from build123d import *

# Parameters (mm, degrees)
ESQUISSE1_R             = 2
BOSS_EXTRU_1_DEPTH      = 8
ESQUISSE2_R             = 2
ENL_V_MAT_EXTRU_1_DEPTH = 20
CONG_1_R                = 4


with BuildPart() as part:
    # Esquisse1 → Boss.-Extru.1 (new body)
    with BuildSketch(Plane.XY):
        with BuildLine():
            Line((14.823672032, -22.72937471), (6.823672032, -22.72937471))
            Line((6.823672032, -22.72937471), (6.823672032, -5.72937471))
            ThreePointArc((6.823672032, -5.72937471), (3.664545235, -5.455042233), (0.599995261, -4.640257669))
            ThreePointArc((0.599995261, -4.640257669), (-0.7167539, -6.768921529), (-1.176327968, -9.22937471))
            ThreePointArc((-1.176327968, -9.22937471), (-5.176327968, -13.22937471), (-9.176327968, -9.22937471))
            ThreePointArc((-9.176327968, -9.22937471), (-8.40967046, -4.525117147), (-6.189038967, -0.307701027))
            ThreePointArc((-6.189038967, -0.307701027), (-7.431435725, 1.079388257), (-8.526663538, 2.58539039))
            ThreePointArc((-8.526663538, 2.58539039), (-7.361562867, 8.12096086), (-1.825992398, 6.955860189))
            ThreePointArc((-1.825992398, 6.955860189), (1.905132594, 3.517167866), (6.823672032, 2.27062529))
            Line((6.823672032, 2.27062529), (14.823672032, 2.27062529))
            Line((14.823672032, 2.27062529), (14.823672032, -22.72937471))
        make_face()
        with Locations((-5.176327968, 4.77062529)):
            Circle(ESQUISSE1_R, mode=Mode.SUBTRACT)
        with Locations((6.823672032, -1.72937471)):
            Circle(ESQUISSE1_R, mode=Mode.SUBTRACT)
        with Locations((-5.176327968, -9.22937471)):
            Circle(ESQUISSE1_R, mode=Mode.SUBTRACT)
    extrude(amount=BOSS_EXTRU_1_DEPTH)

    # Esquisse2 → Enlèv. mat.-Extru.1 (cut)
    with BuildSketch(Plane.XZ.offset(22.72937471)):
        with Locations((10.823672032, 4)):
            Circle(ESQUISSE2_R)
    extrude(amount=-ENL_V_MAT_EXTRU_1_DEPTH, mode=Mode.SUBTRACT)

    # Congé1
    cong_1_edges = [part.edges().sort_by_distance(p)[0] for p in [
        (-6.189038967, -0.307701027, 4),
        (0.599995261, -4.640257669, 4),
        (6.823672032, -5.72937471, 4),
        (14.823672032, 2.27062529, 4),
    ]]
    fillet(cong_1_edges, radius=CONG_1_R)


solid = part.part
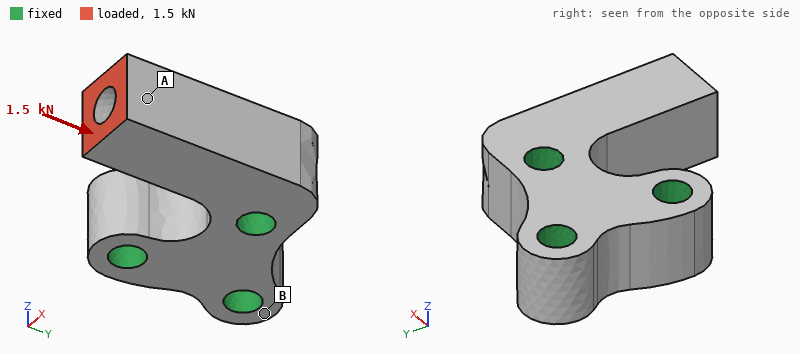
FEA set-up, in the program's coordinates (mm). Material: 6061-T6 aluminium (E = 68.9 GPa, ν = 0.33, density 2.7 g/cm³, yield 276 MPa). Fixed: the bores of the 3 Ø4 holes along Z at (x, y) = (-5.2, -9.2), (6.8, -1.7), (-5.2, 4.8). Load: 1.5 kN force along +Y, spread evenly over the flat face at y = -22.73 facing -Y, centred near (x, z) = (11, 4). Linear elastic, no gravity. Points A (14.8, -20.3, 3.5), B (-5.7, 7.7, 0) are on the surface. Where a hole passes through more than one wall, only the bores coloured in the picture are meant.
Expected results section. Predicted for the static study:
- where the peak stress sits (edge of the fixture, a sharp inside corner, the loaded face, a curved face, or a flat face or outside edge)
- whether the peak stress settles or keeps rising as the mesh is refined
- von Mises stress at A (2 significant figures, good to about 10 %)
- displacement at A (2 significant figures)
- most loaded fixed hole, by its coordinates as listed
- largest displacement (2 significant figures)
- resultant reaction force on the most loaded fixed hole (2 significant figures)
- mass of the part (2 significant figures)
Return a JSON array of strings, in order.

["edge of the fixture", "keeps rising", "29 MPa", "24 µm", "(6.8, -1.7)", "27 µm", "1.6 kN", "7.7 g"]
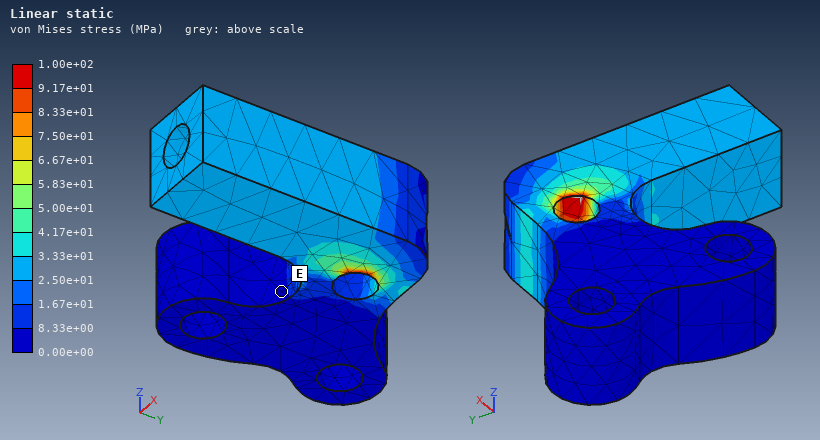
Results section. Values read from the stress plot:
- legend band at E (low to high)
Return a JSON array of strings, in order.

["0.00e+00 to 8.33e+00 MPa"]
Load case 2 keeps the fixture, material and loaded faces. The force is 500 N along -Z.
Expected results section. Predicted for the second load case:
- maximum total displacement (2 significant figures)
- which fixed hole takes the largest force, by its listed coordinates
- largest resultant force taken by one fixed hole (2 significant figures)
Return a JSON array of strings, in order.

["80 µm", "(6.8, -1.7)", "530 N"]
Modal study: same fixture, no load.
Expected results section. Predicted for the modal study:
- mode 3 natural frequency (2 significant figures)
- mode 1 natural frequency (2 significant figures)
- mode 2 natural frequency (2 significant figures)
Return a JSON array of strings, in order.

["35 kHz", "14 kHz", "14 kHz"]
